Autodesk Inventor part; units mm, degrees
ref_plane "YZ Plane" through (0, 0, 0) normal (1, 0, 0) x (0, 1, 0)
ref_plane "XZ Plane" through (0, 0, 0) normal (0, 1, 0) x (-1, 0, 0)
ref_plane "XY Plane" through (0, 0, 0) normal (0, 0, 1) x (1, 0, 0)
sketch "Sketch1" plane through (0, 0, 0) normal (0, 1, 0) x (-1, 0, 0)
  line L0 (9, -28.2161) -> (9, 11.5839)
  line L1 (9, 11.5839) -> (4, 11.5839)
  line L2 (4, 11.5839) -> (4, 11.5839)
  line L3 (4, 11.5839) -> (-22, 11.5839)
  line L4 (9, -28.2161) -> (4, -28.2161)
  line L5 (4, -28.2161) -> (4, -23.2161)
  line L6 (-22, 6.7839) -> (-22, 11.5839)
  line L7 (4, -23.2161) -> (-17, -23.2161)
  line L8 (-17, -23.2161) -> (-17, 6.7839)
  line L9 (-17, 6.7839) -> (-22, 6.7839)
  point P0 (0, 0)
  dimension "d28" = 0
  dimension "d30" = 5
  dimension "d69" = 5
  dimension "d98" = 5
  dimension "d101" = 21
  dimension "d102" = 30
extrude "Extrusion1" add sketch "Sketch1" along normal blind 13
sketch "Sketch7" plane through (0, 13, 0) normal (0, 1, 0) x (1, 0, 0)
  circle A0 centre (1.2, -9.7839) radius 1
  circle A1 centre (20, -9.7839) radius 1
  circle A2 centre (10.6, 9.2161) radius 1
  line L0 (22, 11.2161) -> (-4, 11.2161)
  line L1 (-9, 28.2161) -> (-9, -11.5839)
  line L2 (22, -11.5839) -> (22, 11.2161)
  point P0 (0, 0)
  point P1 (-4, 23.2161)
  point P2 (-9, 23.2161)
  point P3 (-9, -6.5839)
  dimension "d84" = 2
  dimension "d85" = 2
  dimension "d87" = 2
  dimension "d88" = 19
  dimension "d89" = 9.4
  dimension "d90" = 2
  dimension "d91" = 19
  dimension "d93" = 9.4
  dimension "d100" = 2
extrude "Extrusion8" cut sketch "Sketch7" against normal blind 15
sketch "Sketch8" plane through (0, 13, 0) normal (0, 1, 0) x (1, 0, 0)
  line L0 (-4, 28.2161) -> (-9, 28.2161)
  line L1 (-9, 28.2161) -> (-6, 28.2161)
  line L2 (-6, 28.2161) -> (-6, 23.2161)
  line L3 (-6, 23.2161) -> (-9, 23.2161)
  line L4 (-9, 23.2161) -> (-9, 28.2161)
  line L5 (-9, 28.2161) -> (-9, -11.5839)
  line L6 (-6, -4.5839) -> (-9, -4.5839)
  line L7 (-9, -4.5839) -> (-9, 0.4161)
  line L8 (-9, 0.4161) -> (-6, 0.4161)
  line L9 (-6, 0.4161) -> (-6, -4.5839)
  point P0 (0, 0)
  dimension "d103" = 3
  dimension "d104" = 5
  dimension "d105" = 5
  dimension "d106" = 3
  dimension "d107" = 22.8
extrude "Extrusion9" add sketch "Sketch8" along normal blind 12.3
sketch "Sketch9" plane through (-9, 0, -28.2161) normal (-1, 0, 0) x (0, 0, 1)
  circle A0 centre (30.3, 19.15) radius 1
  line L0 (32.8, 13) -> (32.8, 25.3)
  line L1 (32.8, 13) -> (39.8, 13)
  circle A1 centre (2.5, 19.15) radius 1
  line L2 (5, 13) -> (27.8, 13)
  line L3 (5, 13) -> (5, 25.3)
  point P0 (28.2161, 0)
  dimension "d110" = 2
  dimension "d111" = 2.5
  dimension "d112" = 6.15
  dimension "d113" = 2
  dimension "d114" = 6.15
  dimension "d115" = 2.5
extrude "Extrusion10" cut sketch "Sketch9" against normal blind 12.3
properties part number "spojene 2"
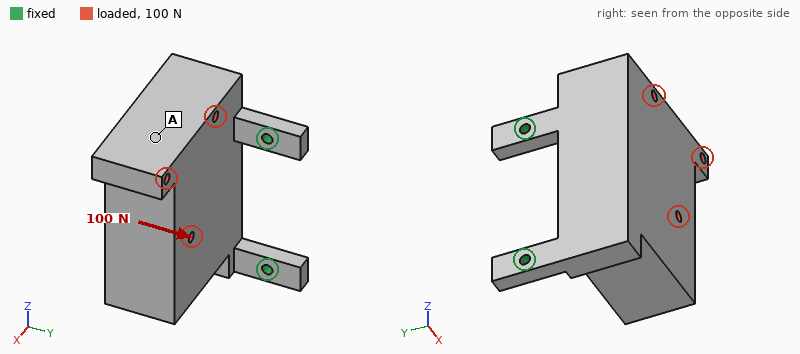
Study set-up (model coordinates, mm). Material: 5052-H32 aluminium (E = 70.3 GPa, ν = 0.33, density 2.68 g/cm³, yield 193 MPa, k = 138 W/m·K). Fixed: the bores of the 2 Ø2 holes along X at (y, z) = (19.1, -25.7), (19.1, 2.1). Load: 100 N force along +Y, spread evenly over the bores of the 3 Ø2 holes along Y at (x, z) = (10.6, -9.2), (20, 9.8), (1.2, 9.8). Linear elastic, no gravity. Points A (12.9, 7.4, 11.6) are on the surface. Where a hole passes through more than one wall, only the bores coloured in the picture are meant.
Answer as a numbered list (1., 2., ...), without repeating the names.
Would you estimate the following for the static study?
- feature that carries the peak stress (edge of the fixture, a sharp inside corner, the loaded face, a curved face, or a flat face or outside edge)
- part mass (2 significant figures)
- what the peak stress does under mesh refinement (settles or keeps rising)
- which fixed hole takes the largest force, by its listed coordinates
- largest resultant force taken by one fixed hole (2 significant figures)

1. edge of the fixture
2. 34 g
3. keeps rising
4. (19.1, 2.1)
5. 100 N
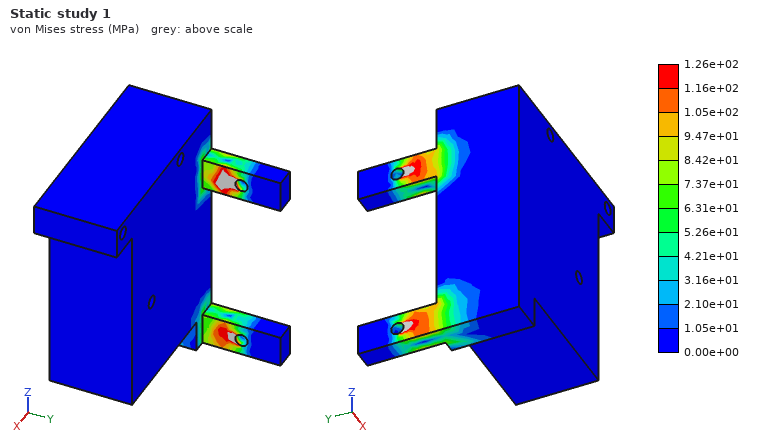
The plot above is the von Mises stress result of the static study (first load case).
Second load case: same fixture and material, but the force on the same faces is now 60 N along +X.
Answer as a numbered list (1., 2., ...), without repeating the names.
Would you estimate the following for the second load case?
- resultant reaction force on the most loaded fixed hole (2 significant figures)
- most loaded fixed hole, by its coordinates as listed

1. 62 N
2. (19.1, 2.1)
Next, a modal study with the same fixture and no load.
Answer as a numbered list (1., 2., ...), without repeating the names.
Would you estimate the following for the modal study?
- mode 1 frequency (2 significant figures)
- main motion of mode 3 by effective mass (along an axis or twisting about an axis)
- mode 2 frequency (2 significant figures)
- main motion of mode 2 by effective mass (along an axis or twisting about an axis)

1. 780 Hz
2. along X
3. 3500 Hz
4. along Z
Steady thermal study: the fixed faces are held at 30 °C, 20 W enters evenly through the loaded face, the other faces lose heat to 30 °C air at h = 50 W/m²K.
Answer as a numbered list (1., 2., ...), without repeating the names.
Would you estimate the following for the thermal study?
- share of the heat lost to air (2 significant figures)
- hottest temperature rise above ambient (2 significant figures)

1. 29 %
2. 39 K
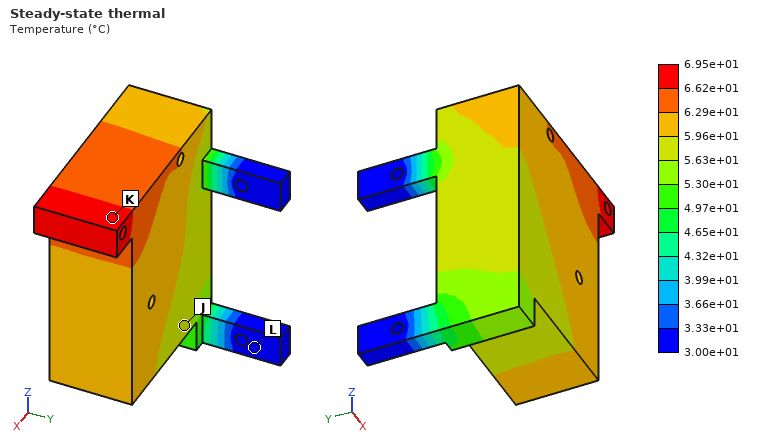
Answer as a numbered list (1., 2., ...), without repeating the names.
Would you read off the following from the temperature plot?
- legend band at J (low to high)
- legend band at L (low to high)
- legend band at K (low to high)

1. 5.63e+01 to 5.96e+01 °C
2. 3.00e+01 to 3.33e+01 °C
3. 6.62e+01 to 6.95e+01 °C
